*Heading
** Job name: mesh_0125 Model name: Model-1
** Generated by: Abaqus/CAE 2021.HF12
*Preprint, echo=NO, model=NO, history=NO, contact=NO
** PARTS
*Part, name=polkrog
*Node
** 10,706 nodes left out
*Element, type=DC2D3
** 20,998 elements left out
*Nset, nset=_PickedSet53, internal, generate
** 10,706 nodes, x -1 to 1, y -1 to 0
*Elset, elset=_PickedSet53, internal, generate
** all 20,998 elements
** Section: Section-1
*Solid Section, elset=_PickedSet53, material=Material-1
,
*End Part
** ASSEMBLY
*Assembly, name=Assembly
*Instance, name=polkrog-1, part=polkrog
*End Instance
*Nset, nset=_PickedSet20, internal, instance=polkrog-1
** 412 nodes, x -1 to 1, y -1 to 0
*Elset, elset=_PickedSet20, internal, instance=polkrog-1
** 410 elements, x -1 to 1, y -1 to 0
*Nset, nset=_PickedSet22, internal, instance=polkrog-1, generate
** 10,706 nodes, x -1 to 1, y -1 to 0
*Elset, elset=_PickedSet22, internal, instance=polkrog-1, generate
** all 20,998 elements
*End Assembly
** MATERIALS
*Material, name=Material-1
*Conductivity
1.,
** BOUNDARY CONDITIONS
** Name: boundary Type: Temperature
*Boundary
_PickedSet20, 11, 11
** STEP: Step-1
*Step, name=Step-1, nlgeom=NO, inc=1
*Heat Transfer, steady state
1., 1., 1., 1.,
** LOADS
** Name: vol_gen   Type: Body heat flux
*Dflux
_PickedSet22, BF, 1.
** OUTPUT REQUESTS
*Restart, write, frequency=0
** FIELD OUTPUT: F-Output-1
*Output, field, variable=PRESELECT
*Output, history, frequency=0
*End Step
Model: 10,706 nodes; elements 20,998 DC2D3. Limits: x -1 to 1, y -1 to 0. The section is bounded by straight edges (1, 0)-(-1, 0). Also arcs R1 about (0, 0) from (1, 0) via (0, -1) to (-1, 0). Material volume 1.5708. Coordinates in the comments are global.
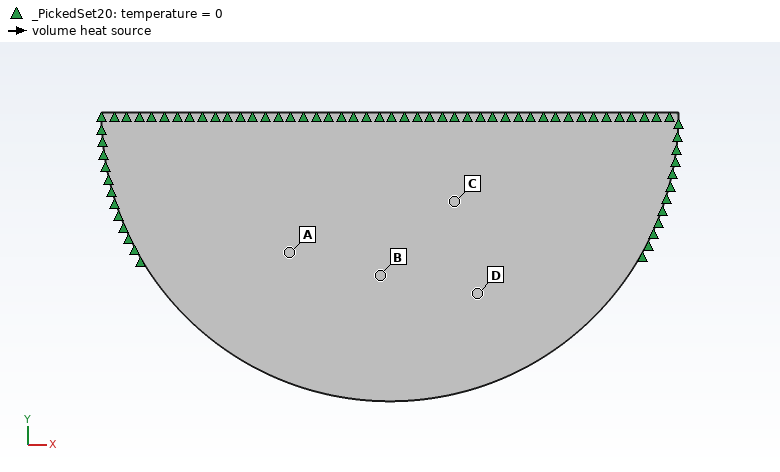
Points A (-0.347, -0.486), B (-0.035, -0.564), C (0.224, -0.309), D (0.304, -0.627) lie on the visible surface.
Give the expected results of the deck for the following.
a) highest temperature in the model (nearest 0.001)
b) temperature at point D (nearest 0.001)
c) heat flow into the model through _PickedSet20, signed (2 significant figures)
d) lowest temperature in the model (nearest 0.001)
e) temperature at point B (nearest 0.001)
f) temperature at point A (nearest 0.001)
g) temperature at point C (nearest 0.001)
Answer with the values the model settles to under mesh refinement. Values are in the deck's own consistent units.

0.098
0.077
-1.6
0.000
0.095
0.084
0.082
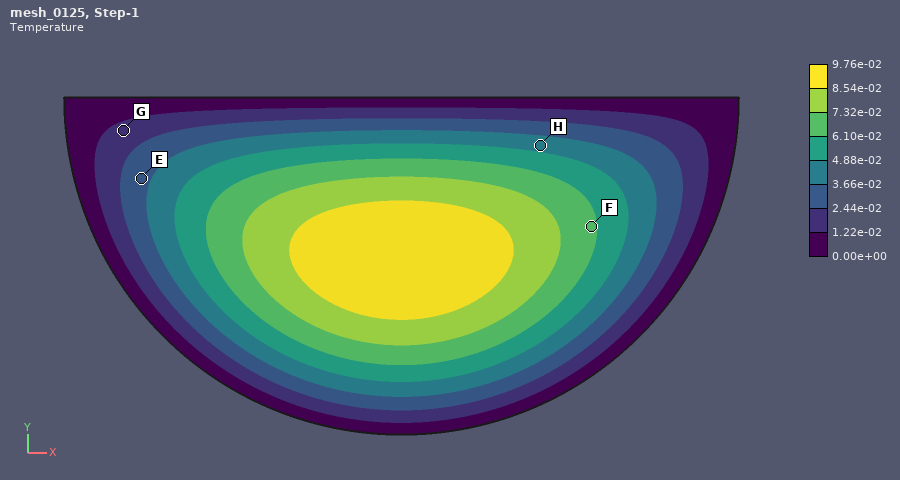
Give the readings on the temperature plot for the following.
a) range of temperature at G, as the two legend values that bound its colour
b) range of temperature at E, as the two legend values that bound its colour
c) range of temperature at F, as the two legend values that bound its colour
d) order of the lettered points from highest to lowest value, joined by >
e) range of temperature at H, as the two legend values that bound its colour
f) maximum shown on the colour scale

1.22e-02 to 2.44e-02
2.44e-02 to 3.66e-02
6.10e-02 to 7.32e-02
F > H > E > G
3.66e-02 to 4.88e-02
9.76e-02
